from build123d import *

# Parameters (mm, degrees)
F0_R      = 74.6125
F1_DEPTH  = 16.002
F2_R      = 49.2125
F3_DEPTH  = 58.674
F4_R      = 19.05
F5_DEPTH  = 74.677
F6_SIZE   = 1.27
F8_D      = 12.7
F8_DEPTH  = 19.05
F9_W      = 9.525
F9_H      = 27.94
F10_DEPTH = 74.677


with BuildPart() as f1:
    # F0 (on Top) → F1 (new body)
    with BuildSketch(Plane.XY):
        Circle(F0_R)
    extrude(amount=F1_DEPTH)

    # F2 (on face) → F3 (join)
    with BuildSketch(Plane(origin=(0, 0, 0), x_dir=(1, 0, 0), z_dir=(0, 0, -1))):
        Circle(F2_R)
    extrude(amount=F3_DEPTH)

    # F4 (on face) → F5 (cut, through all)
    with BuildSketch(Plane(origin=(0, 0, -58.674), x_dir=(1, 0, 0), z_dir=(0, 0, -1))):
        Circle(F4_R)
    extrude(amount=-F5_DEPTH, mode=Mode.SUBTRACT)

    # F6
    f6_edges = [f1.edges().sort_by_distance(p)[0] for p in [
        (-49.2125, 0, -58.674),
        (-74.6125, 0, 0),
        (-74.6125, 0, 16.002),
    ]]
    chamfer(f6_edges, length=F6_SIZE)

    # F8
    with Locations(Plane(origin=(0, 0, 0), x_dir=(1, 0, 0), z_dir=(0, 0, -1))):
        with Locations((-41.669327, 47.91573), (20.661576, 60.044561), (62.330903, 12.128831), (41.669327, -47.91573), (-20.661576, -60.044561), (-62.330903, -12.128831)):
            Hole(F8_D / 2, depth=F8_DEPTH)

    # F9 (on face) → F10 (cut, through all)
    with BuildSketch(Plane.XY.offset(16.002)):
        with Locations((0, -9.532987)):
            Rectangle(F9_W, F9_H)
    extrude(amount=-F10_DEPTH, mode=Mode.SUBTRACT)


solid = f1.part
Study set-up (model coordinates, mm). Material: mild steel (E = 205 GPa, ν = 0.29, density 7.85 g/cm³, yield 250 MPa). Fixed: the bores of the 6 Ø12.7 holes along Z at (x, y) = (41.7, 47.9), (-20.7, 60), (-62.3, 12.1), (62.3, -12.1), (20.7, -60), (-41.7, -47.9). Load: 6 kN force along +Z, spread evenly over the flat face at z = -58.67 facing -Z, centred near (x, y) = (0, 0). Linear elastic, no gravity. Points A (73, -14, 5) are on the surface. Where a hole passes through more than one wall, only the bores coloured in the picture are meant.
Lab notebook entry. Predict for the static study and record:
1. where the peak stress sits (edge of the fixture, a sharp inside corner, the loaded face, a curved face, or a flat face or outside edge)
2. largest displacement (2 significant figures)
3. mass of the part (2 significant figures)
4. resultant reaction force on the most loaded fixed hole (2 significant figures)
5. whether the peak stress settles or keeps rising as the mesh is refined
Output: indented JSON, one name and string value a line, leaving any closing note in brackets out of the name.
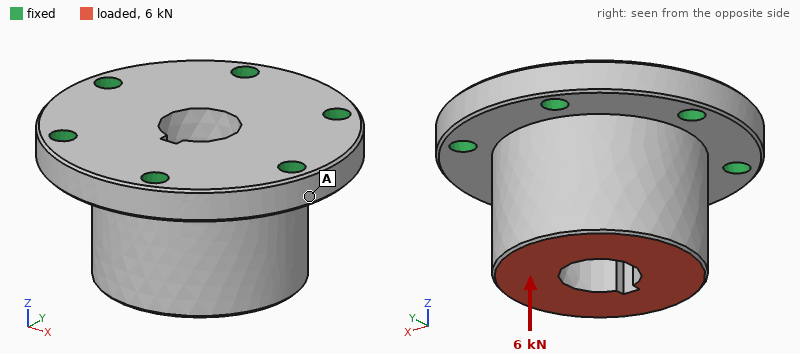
{
  "where the peak stress sits": "edge of the fixture",
  "largest displacement": "0.93 µm",
  "mass of the part": "4.9 kg",
  "resultant reaction force on the most loaded fixed hole": "1.1 kN",
  "whether the peak stress settles or keeps rising as the mesh is refined": "keeps rising"
}
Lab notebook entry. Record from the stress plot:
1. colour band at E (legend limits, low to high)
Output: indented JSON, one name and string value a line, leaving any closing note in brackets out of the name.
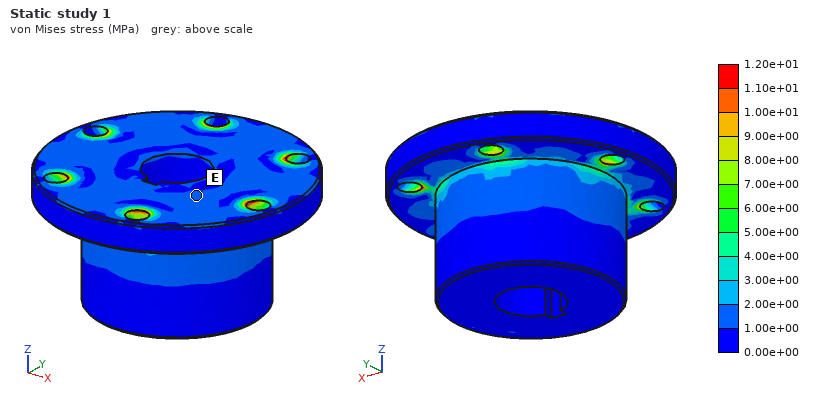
{
  "colour band at E": "1.00e+00 to 2.00e+00 MPa"
}
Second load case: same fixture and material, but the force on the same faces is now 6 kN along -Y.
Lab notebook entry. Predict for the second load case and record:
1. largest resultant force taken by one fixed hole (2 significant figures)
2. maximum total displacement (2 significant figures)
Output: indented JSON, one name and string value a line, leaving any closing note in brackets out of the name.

{
  "largest resultant force taken by one fixed hole": "2.6 kN",
  "maximum total displacement": "3.9 µm"
}
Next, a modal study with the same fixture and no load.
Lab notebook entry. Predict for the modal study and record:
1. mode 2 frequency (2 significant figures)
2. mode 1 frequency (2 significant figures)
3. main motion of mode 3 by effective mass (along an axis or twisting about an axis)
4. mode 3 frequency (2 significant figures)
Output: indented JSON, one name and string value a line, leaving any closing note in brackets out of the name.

{
  "mode 2 frequency": "5900 Hz",
  "mode 1 frequency": "5800 Hz",
  "main motion of mode 3 by effective mass": "along Z",
  "mode 3 frequency": "7200 Hz"
}
